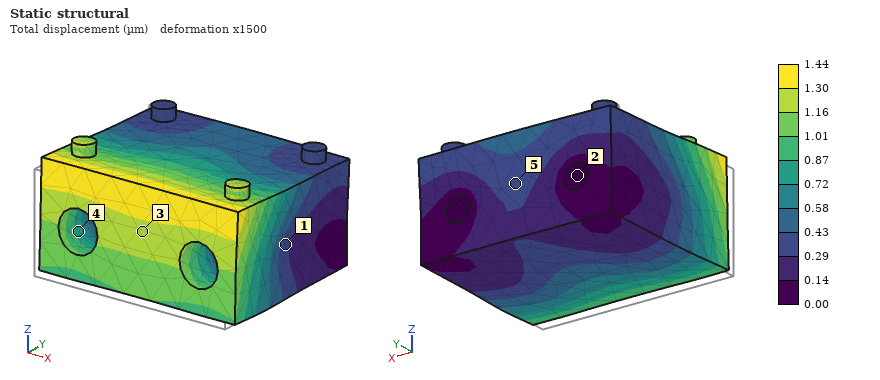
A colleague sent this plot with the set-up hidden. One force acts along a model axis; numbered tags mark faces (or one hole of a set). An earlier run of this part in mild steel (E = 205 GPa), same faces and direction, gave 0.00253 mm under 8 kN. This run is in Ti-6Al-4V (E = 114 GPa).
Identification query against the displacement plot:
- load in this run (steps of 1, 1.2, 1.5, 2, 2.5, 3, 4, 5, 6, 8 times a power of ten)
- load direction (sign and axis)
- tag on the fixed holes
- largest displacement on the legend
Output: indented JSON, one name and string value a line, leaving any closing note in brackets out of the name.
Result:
{
  "load in this run": "2.5 kN",
  "load direction": "+Y",
  "tag on the fixed holes": "2",
  "largest displacement on the legend": "1.44 µm"
}
